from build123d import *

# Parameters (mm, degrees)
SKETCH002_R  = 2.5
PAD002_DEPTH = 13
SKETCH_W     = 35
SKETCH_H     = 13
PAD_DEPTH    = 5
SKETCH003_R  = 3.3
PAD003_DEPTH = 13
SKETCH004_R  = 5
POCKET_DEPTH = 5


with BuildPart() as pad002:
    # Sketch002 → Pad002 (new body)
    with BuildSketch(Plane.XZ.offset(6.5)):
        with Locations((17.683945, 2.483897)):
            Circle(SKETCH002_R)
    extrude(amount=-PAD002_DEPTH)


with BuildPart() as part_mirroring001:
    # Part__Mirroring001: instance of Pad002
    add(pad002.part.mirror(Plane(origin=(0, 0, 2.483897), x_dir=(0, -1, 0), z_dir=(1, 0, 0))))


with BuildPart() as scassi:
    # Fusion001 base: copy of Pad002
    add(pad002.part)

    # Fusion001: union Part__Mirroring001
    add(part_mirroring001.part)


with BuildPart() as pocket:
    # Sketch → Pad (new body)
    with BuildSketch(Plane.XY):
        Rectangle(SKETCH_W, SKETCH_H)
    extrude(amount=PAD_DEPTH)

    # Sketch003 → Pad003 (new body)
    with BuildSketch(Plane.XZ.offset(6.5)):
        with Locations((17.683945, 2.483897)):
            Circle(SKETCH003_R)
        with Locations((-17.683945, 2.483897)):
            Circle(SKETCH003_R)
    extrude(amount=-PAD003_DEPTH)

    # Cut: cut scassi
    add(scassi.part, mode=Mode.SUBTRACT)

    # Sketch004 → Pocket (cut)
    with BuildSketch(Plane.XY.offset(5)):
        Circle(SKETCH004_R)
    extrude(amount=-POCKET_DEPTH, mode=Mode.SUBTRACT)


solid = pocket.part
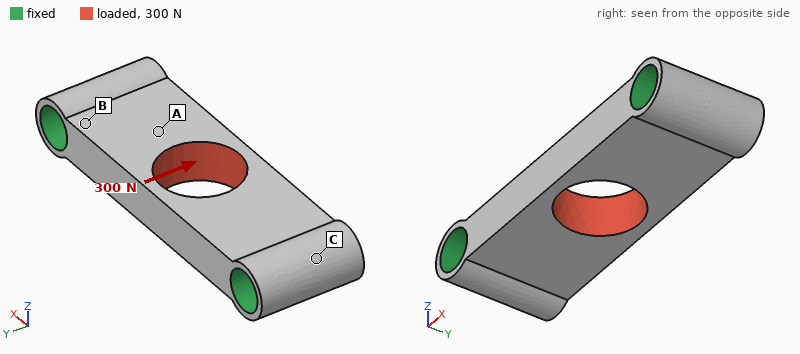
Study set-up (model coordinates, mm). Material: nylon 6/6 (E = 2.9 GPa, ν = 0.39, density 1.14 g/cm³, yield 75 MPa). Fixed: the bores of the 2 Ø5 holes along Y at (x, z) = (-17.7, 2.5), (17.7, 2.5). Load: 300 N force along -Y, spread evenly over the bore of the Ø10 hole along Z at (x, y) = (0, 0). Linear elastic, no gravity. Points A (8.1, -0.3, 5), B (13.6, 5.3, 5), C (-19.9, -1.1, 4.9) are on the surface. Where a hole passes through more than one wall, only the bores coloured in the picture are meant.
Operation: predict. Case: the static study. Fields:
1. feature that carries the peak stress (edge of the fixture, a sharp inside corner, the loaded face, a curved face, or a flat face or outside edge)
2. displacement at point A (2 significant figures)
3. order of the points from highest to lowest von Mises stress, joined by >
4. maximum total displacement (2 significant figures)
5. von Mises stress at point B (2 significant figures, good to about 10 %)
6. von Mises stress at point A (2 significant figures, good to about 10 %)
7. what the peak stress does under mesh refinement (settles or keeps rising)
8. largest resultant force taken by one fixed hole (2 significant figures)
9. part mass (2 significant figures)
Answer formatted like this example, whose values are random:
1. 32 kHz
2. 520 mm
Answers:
1. edge of the fixture
2. 27 µm
3. A > B > C
4. 66 µm
5. 4.6 MPa
6. 7.0 MPa
7. keeps rising
8. 150 N
9. 2.2 g
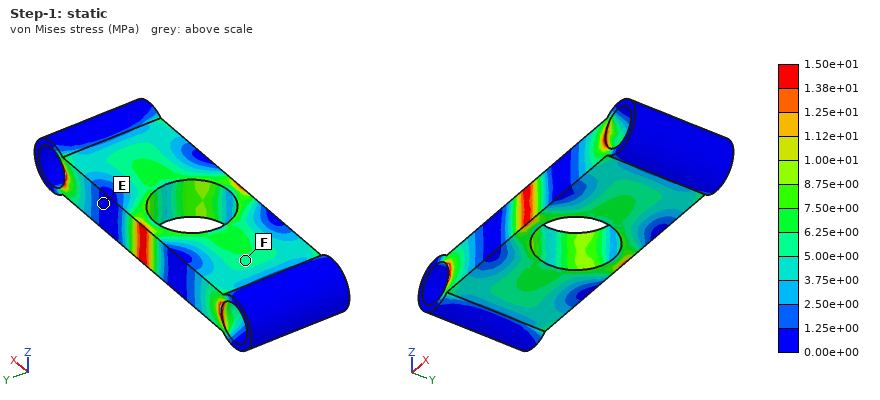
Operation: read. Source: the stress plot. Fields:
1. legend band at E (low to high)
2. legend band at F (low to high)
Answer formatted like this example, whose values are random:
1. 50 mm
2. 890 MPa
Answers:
1. 0.00e+00 to 1.25e+00 MPa
2. 5.00e+00 to 6.25e+00 MPa
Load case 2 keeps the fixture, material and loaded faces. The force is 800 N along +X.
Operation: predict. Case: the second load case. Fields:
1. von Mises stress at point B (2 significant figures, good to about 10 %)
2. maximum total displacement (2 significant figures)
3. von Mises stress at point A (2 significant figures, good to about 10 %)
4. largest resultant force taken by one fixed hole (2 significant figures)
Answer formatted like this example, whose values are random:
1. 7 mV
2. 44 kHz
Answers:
1. 5.2 MPa
2. 36 µm
3. 5.6 MPa
4. 400 N
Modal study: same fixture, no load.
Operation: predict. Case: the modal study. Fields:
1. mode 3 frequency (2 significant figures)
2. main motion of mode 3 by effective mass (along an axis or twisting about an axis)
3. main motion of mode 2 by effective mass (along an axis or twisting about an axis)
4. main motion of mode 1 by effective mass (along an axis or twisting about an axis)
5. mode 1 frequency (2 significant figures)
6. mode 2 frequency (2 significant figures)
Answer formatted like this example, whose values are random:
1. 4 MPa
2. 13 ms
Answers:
1. 15 kHz
2. along Y
3. twisting about X
4. along Z
5. 8000 Hz
6. 11 kHz
